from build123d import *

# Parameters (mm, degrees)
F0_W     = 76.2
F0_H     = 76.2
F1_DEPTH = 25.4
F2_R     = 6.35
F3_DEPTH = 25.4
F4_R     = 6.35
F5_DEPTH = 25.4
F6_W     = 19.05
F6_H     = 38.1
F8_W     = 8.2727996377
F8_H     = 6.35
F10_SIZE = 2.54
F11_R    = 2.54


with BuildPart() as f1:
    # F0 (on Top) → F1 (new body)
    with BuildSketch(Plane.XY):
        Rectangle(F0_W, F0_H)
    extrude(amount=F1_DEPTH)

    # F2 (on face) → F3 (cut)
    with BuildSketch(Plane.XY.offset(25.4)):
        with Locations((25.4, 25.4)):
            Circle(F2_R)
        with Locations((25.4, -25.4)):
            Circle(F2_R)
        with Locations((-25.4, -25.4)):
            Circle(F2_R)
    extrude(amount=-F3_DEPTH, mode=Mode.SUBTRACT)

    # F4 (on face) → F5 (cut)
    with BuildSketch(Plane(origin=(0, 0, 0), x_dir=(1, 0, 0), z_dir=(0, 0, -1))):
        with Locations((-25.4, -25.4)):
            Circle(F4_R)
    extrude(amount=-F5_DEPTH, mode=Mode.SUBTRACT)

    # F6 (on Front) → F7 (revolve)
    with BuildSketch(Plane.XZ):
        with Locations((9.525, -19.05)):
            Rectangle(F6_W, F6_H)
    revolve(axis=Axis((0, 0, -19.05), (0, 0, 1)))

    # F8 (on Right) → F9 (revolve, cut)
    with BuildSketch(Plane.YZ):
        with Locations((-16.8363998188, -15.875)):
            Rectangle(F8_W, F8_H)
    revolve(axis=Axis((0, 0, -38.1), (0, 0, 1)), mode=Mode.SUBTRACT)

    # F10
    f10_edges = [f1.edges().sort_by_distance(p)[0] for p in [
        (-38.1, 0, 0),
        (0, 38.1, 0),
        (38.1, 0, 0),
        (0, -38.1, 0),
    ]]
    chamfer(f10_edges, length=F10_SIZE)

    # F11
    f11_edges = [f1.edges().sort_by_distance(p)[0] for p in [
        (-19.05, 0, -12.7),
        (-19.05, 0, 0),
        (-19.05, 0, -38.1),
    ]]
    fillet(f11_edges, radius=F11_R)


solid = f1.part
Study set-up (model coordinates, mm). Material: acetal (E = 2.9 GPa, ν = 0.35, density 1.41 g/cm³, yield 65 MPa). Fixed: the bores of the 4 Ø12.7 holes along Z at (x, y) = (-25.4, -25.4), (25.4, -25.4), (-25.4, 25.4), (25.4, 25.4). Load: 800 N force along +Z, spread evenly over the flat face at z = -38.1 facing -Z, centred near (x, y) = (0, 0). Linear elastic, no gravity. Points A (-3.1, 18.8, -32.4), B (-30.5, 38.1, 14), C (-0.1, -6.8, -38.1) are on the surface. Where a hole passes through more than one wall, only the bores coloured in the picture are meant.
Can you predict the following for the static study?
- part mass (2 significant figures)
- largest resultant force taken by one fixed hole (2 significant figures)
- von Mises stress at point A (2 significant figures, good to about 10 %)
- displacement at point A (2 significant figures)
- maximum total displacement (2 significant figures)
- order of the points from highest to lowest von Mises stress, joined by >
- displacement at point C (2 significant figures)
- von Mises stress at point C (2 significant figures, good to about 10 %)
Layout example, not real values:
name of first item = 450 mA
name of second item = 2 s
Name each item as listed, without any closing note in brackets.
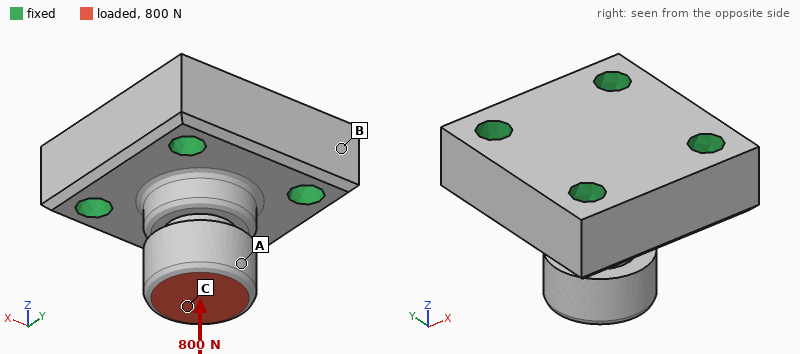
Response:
part mass = 240 g
largest resultant force taken by one fixed hole = 210 N
von Mises stress at point A = 0.36 MPa
displacement at point A = 19 µm
maximum total displacement = 21 µm
order of the points from highest to lowest von Mises stress, joined by > = C > A > B
displacement at point C = 21 µm
von Mises stress at point C = 0.90 MPa
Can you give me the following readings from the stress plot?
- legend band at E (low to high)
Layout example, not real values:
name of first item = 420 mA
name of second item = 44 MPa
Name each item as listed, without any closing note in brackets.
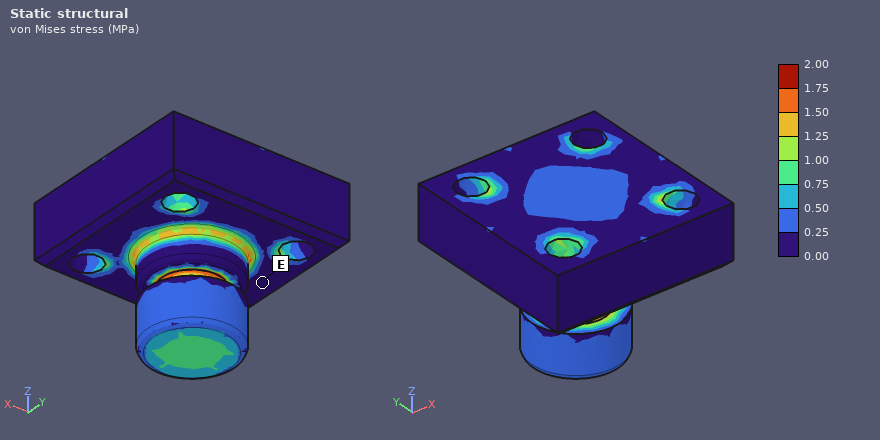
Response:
legend band at E = 0.00 to 0.25 MPa
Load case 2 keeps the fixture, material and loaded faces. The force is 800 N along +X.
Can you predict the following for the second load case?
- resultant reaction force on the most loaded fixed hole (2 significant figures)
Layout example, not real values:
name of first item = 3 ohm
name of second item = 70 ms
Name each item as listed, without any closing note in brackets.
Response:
resultant reaction force on the most loaded fixed hole = 470 N
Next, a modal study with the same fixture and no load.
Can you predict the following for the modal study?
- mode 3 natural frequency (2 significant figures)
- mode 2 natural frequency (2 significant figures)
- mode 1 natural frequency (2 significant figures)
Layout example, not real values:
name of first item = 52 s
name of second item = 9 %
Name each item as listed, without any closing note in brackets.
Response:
mode 3 natural frequency = 3600 Hz
mode 2 natural frequency = 2300 Hz
mode 1 natural frequency = 2300 Hz
